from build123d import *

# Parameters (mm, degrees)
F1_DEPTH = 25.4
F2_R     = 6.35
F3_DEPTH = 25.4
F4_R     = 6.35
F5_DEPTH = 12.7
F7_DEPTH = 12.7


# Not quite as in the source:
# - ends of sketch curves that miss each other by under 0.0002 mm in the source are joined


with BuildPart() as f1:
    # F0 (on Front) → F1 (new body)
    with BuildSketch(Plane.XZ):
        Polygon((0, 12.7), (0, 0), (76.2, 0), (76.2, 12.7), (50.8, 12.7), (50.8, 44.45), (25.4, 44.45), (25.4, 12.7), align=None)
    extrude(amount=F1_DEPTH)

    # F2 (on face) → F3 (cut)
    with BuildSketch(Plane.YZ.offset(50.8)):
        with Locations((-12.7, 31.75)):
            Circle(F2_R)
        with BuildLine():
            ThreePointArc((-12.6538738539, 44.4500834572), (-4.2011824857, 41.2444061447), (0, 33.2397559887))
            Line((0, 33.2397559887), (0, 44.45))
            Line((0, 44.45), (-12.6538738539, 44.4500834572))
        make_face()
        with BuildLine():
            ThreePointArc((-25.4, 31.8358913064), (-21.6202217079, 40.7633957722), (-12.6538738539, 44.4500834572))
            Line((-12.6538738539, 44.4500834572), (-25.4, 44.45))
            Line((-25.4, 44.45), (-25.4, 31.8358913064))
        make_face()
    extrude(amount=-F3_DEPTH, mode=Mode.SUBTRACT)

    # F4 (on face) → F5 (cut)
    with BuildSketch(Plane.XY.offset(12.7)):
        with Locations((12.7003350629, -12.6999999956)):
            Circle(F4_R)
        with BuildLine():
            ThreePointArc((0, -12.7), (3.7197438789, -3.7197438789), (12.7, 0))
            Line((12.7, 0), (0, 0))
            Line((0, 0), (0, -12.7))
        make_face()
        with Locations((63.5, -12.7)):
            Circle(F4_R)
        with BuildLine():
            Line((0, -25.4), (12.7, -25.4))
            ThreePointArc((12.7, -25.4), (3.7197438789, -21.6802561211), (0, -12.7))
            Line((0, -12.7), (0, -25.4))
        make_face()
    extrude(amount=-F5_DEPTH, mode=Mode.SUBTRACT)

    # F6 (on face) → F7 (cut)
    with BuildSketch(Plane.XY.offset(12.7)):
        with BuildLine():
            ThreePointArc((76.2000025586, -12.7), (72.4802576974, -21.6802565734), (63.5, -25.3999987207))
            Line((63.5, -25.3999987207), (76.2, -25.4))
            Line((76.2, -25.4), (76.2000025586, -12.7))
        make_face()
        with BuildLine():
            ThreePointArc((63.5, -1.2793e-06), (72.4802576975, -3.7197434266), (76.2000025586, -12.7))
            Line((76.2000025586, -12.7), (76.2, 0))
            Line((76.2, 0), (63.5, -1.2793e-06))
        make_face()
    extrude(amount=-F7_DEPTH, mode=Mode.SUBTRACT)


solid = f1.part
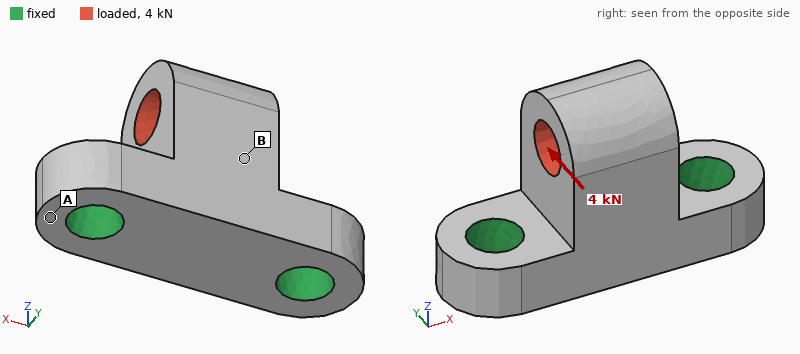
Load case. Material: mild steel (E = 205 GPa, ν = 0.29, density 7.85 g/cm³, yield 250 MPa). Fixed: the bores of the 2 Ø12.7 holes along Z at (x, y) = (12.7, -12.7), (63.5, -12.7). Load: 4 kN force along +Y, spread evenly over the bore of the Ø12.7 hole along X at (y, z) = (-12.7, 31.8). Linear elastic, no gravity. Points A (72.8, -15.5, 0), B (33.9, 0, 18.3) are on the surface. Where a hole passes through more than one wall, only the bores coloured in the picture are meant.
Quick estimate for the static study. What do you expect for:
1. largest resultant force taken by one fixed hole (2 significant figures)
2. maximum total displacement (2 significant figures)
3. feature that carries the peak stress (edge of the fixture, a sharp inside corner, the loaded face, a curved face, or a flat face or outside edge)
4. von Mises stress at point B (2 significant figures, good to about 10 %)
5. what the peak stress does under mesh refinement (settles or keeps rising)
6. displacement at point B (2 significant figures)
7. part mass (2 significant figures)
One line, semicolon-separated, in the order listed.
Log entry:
2.0 kN; 29 µm; edge of the fixture; 20 MPa; keeps rising; 12 µm; 280 g
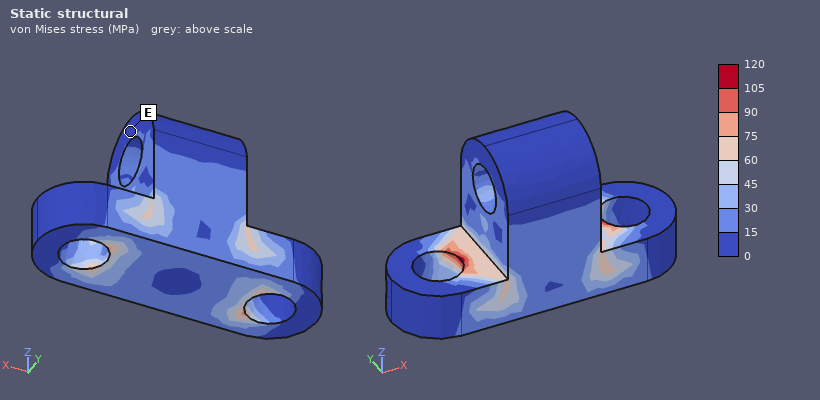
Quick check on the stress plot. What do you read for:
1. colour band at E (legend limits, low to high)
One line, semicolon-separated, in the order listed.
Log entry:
0 to 15 MPa
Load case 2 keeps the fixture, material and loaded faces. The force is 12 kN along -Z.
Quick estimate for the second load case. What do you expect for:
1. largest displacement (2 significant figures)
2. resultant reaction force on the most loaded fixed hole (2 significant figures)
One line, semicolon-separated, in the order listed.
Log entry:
9.2 µm; 6.3 kN
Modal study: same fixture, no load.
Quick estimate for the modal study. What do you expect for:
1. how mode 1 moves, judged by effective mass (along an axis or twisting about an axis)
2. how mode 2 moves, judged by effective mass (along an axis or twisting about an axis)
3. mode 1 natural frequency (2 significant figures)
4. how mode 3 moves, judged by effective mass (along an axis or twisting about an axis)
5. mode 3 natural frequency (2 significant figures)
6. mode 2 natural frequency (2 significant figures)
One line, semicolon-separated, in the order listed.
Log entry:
along Y; along X; 7100 Hz; along Z; 17 kHz; 12 kHz
